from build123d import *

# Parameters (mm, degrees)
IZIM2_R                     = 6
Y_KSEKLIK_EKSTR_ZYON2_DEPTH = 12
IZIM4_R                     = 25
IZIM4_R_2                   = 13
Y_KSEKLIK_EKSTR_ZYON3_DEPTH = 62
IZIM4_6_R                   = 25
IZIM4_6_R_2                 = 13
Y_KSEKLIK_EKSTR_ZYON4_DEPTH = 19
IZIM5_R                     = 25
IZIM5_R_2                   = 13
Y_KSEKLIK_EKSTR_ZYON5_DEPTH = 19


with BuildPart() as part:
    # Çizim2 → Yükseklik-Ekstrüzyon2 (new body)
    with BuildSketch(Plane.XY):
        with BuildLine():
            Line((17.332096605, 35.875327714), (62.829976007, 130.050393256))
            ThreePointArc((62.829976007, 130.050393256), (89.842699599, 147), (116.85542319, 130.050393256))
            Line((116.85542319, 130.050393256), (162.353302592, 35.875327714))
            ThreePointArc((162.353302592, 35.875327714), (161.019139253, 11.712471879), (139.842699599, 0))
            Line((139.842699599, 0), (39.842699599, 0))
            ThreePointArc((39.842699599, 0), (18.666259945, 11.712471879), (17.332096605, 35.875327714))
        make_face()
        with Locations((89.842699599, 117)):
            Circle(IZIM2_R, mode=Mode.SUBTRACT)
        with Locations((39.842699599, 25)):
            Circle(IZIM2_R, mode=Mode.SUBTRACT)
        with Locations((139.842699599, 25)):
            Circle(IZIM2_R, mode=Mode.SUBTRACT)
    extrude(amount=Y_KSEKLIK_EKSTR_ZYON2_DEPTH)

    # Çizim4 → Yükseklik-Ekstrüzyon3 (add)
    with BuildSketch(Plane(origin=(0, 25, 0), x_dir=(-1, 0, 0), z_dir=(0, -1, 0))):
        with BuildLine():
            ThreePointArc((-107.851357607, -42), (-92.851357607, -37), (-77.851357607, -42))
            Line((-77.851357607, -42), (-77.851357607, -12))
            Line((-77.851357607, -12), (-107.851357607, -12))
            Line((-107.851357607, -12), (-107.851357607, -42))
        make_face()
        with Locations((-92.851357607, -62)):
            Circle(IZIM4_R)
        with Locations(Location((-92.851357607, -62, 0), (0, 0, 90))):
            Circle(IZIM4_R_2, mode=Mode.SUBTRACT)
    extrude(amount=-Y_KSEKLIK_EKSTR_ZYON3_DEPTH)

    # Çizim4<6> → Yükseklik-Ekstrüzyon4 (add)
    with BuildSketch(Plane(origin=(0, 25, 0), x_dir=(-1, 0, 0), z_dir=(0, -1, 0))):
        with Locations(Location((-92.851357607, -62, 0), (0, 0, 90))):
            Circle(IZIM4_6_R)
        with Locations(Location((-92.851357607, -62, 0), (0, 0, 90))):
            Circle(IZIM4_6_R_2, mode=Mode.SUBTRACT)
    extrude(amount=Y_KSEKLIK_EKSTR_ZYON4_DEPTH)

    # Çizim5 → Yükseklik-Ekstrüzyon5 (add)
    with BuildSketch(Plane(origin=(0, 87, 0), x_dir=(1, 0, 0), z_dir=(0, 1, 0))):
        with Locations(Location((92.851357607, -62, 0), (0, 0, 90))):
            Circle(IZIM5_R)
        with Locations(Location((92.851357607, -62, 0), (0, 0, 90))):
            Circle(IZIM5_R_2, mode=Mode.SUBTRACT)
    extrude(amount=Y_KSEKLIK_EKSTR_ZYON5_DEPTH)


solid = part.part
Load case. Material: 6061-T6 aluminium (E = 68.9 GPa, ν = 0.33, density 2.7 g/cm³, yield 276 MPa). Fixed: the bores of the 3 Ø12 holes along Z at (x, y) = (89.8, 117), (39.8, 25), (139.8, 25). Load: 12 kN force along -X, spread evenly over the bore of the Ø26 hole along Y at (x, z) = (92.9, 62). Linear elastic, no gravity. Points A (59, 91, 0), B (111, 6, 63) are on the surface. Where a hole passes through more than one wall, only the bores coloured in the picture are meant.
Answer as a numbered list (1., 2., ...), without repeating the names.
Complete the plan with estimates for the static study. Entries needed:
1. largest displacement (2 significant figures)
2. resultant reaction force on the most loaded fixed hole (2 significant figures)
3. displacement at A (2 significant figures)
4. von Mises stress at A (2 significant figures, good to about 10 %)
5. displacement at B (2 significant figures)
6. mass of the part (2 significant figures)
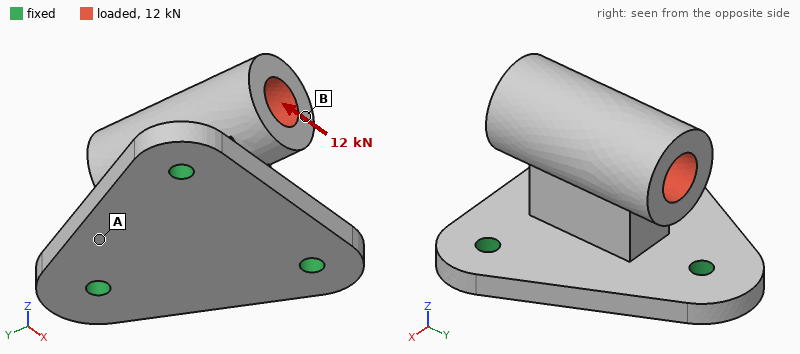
1. 0.40 mm
2. 9.0 kN
3. 0.060 mm
4. 30 MPa
5. 0.27 mm
6. 1000 g
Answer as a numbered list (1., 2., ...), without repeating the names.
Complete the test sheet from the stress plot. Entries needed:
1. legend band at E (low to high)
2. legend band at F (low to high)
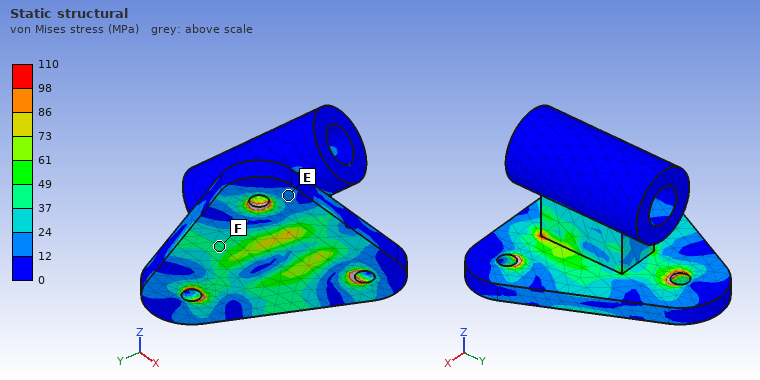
1. 12 to 24 MPa
2. 37 to 49 MPa
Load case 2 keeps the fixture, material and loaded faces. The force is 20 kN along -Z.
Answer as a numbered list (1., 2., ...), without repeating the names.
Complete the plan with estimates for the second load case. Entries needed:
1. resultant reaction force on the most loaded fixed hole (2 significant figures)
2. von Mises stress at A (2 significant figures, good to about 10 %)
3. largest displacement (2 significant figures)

1. 7.4 kN
2. 26 MPa
3. 0.10 mm
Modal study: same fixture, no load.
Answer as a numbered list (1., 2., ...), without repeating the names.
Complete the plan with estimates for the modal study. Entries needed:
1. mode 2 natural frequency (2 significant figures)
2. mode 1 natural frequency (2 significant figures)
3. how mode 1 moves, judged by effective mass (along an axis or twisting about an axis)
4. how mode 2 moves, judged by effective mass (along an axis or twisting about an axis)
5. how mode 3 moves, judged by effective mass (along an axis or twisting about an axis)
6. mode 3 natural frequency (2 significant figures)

1. 2000 Hz
2. 1600 Hz
3. along X
4. along Y
5. along Z
6. 3000 Hz
